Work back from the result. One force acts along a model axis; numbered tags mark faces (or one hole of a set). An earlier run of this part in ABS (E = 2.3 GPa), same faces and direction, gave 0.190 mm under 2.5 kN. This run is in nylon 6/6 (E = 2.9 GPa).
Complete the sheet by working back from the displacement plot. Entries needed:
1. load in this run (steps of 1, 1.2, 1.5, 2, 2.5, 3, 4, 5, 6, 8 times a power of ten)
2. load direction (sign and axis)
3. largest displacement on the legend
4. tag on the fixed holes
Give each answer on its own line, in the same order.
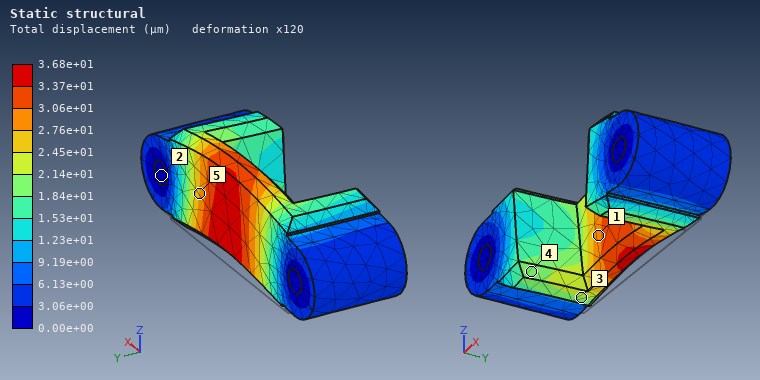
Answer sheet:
600 N
+Z
3.68e+01 µm
2
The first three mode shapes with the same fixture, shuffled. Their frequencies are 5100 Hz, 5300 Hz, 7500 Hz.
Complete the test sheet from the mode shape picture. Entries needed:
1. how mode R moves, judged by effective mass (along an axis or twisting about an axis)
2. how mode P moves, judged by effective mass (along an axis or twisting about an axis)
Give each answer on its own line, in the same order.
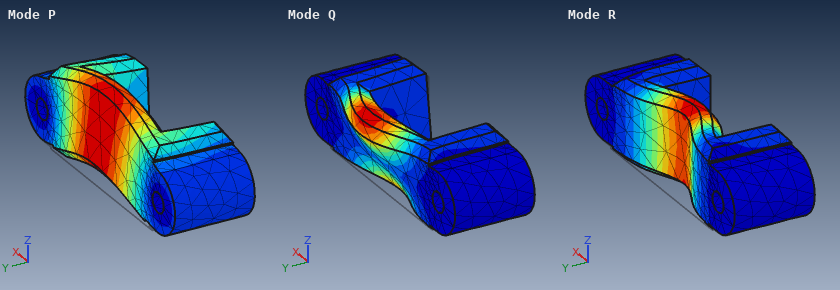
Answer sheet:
along Y
along Z
